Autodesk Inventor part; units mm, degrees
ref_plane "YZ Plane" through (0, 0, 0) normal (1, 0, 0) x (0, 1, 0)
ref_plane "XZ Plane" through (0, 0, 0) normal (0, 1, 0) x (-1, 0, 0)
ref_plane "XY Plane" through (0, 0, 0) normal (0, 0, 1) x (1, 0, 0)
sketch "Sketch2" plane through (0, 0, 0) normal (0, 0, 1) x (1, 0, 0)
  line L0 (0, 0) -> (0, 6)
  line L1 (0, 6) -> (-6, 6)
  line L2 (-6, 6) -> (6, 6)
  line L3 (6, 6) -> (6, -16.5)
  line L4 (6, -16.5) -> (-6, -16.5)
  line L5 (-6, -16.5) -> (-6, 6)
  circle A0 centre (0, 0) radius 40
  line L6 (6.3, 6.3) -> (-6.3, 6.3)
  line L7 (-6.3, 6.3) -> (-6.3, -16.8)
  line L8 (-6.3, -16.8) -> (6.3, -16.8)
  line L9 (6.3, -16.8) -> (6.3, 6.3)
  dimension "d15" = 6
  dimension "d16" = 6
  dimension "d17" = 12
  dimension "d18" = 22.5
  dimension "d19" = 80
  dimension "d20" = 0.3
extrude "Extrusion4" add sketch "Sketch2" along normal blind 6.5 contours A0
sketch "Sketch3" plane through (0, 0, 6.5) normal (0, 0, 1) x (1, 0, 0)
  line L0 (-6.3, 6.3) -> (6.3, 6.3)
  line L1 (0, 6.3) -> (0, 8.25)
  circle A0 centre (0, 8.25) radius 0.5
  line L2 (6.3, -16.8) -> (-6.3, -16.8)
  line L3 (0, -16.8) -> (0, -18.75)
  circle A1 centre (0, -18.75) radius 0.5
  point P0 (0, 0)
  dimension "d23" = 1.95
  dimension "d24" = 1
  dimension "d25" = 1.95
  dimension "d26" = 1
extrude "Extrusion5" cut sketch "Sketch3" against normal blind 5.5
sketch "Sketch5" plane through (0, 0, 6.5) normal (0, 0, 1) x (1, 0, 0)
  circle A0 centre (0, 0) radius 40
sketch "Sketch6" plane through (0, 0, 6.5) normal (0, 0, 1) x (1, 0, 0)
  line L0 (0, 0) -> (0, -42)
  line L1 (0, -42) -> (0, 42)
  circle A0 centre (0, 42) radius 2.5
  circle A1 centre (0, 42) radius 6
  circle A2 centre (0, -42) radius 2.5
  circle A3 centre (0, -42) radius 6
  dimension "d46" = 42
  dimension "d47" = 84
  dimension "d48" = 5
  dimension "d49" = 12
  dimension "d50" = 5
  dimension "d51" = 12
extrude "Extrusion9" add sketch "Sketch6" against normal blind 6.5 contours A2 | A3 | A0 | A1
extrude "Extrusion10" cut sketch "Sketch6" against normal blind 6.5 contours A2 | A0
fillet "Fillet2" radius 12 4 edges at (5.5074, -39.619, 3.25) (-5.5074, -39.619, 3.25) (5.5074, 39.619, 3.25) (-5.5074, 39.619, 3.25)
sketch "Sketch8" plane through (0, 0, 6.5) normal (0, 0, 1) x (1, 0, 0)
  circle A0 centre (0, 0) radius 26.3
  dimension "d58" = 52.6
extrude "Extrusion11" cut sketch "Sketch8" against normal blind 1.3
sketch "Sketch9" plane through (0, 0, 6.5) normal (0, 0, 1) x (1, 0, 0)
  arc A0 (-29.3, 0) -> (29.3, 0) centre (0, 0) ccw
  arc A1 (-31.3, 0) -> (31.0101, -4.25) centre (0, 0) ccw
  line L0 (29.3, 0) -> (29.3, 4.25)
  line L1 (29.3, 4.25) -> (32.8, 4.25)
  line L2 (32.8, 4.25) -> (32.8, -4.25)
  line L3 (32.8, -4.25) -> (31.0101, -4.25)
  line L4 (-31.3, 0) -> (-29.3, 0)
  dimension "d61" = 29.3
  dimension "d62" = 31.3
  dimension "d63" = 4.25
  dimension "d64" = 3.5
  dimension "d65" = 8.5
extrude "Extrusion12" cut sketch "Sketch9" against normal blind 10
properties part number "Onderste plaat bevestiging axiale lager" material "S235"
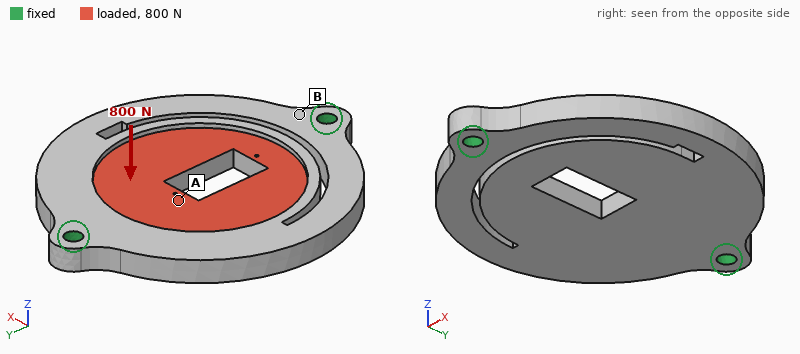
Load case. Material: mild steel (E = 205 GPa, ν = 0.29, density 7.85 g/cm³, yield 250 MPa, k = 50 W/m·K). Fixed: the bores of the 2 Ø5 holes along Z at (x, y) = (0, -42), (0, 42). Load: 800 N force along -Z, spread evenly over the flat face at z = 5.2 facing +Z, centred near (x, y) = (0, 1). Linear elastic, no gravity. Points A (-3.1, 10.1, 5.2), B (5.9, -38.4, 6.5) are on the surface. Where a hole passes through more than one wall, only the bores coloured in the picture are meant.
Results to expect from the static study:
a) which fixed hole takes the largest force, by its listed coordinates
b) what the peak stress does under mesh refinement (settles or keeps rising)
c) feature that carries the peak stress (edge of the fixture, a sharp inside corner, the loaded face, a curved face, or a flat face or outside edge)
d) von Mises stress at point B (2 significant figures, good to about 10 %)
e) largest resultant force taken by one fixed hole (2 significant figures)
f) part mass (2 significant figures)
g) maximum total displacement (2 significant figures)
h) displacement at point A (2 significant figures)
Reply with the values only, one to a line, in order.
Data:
(0, 42)
keeps rising
edge of the fixture
38 MPa
500 N
220 g
0.12 mm
0.041 mm
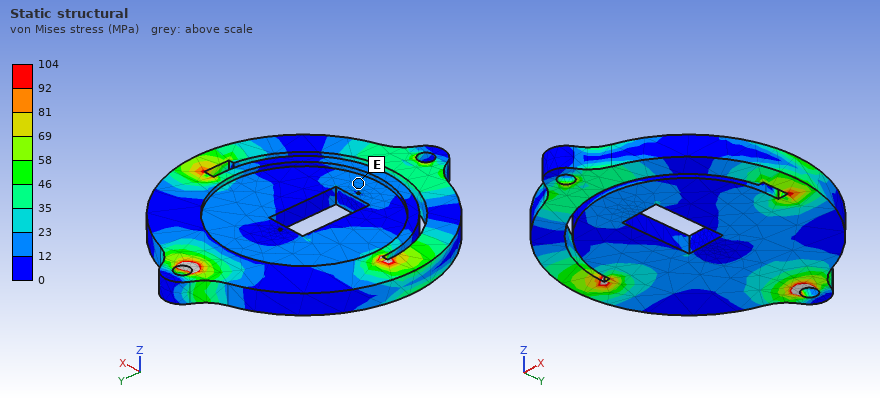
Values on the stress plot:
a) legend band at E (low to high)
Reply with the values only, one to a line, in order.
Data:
12 to 23 MPa
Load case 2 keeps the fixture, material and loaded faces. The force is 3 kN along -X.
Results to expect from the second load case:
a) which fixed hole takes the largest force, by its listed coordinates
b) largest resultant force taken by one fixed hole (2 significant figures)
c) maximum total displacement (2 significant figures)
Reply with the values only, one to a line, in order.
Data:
(0, 42)
1.8 kN
36 µm
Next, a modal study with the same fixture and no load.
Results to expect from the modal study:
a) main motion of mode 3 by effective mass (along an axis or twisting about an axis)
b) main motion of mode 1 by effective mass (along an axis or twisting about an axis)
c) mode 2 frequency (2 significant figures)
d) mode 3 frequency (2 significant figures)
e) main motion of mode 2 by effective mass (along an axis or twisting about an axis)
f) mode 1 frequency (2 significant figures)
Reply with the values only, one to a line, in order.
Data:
along Z
along Z
1800 Hz
3400 Hz
twisting about Y
1500 Hz
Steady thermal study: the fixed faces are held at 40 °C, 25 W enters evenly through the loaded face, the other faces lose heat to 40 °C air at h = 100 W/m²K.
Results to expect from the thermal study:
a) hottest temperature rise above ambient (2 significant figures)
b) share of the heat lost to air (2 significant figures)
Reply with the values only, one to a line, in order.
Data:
32 K
69 %
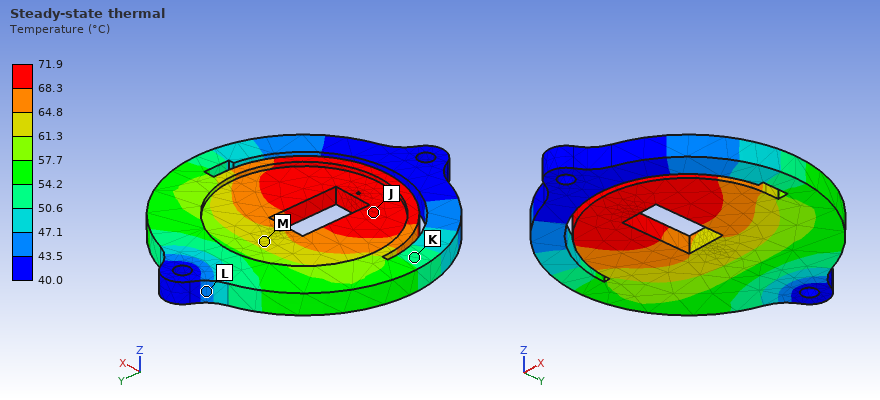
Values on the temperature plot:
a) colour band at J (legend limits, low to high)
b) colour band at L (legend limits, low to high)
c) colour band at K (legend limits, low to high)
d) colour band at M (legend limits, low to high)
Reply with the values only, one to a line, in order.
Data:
68.3 to 71.9 °C
43.5 to 47.1 °C
50.6 to 54.2 °C
61.3 to 64.8 °C
